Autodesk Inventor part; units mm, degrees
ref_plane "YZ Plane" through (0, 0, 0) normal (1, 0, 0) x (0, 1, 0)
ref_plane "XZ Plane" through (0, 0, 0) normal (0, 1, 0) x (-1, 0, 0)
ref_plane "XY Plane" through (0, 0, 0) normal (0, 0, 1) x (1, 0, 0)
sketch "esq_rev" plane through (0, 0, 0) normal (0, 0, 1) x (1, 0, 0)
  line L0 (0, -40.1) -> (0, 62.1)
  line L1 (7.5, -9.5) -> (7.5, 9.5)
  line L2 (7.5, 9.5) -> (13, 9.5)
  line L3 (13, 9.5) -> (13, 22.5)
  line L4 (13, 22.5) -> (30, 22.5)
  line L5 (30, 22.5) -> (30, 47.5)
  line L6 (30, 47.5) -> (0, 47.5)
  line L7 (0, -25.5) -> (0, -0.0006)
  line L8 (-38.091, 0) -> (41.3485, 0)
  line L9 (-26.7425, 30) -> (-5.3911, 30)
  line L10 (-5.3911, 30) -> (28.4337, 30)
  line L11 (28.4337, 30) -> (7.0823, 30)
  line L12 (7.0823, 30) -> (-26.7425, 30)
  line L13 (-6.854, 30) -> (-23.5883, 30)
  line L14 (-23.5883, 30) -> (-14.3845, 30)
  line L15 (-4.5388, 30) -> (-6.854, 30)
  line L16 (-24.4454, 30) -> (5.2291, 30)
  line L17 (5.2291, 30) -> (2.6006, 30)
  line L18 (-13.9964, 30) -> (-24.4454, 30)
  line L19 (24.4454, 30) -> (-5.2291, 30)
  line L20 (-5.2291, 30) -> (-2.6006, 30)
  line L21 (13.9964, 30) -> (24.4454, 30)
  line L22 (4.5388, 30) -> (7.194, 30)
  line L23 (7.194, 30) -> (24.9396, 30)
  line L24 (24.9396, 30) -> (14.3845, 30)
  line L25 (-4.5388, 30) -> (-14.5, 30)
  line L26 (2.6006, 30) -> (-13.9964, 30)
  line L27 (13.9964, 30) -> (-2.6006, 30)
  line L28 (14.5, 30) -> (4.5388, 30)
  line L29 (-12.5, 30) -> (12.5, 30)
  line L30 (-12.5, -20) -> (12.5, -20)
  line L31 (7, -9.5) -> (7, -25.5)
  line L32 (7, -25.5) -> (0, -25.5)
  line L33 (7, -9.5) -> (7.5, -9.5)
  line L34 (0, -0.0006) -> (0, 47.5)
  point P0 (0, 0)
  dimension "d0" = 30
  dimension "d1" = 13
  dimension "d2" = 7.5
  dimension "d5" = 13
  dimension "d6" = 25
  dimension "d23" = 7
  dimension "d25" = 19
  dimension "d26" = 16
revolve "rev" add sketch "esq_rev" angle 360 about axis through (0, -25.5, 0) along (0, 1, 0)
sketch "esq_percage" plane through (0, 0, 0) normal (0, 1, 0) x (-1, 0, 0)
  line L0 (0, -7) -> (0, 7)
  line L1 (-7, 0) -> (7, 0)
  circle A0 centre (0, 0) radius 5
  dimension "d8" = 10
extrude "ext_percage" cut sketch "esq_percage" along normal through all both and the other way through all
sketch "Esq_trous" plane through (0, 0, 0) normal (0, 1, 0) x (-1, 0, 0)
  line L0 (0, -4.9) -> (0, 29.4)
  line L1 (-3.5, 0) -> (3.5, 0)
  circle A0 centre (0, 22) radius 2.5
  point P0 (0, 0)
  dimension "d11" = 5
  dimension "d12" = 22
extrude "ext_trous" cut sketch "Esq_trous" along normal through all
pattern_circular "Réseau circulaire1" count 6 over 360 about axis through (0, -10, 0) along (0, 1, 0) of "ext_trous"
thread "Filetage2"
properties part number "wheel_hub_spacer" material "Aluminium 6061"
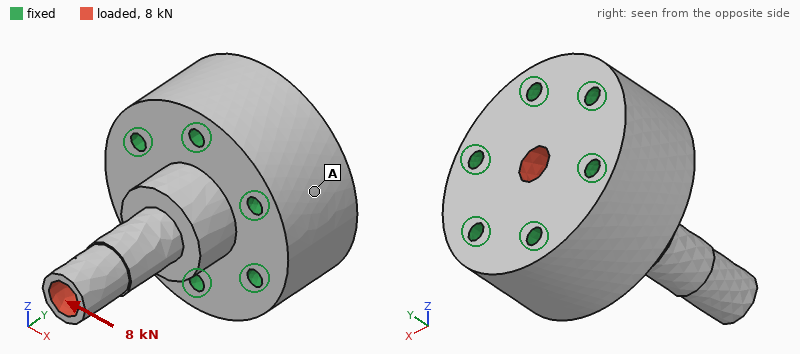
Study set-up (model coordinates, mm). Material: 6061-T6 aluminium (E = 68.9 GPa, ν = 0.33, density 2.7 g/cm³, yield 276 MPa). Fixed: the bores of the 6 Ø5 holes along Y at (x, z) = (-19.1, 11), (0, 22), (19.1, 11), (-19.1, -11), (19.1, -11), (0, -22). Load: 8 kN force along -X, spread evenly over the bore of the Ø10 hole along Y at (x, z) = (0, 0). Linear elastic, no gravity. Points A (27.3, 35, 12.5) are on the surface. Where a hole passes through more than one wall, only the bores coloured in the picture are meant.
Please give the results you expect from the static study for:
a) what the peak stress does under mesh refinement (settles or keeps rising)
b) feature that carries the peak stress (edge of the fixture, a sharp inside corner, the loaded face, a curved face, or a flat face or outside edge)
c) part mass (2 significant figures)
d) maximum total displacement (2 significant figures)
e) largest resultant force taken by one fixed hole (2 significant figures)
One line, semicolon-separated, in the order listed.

keeps rising; a sharp inside corner; 200 g; 0.30 mm; 3.1 kN
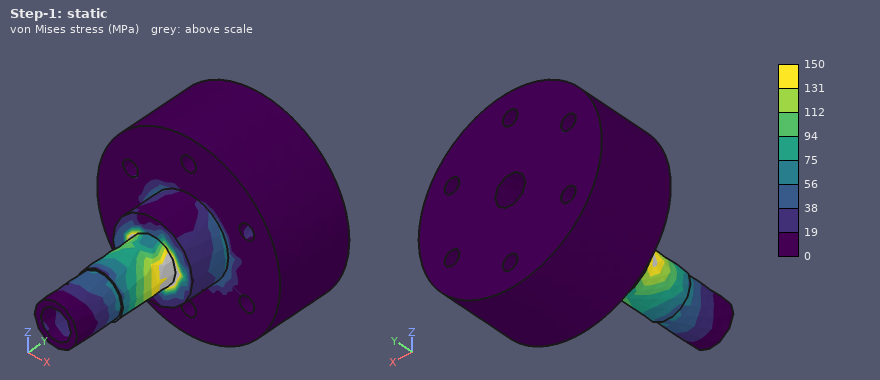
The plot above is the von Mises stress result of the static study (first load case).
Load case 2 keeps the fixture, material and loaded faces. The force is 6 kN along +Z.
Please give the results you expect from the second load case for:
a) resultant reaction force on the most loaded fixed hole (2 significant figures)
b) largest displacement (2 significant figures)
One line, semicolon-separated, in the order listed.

2.7 kN; 0.23 mm
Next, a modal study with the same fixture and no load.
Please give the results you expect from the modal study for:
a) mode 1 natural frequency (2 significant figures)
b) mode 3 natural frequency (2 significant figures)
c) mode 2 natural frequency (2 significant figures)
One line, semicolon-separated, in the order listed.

7900 Hz; 22 kHz; 7900 Hz
